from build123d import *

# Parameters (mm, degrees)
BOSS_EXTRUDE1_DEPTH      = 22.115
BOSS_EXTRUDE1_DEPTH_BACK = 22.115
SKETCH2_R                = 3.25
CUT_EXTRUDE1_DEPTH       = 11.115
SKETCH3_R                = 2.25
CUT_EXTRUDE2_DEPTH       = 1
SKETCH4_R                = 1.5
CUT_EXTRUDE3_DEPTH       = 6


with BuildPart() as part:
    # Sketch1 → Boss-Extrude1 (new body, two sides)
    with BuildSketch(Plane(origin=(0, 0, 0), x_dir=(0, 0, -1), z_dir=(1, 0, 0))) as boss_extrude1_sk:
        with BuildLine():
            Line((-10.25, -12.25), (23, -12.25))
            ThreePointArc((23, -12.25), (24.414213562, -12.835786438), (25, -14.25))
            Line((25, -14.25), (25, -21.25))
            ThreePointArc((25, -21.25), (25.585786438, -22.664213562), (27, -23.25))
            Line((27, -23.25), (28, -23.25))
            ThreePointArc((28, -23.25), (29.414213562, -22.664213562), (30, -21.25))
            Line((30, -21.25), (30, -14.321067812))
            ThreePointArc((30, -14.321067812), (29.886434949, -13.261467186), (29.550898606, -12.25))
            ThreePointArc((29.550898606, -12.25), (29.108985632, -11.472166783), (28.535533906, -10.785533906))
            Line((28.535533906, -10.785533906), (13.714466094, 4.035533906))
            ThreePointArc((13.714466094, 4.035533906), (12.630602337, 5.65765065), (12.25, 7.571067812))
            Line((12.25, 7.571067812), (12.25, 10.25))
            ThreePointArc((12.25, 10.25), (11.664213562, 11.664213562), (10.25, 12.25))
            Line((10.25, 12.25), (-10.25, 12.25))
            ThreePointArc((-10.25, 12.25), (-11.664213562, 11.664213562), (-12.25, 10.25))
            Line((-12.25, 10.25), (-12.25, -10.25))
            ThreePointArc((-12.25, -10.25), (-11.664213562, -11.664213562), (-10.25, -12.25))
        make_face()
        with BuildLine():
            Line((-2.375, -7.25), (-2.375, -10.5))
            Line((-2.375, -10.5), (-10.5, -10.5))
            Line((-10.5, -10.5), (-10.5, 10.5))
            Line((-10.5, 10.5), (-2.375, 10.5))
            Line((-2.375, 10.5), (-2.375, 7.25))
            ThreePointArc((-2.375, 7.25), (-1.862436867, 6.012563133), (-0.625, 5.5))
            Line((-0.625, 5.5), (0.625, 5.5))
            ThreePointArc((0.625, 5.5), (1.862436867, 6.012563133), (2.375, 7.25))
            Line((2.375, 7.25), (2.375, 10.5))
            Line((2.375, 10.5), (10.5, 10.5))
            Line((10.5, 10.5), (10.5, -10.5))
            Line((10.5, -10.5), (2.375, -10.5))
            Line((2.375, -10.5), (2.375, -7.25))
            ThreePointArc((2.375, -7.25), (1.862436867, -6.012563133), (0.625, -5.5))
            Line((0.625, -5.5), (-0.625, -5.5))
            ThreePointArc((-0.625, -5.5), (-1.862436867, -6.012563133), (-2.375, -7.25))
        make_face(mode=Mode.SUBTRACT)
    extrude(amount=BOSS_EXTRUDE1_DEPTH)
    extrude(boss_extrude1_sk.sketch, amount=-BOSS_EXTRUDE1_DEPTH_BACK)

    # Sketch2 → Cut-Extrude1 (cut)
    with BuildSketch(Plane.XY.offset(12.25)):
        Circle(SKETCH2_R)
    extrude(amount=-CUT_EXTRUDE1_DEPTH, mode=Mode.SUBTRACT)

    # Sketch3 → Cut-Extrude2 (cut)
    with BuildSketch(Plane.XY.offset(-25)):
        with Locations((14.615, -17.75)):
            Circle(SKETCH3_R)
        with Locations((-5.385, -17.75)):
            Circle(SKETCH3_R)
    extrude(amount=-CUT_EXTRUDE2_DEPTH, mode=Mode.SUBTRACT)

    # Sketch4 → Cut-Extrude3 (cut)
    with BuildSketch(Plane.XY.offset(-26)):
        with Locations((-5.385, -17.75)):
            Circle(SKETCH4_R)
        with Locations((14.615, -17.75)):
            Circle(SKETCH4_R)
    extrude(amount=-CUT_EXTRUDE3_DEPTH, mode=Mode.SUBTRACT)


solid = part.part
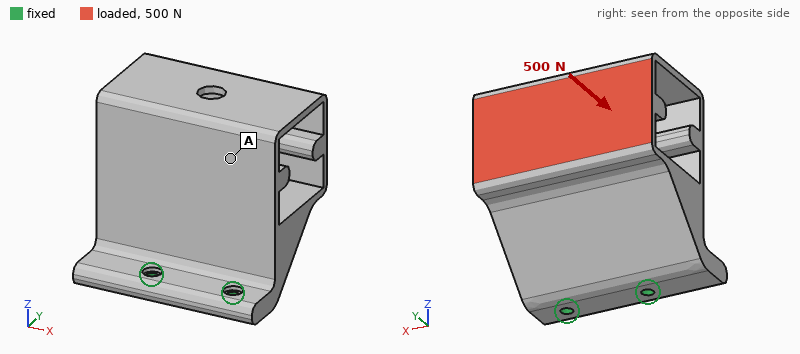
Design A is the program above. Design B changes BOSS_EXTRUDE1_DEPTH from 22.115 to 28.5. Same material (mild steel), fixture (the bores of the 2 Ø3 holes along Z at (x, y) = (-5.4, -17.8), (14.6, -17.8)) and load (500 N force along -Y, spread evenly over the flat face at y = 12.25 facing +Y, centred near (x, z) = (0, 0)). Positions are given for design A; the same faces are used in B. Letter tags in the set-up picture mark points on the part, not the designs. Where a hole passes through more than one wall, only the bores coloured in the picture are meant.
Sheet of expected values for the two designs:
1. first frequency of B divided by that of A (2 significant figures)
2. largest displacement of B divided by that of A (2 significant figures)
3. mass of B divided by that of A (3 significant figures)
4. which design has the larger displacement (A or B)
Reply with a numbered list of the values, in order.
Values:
1. 0.98
2. 0.89
3. 1.15
4. A
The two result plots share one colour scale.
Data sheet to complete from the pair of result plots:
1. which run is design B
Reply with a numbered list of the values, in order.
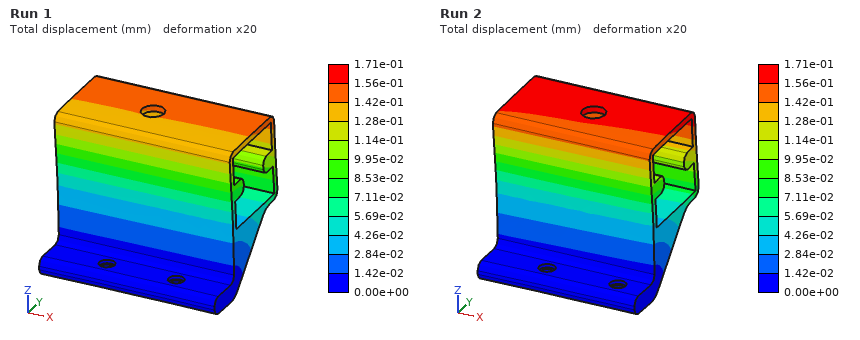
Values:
1. Run 1
